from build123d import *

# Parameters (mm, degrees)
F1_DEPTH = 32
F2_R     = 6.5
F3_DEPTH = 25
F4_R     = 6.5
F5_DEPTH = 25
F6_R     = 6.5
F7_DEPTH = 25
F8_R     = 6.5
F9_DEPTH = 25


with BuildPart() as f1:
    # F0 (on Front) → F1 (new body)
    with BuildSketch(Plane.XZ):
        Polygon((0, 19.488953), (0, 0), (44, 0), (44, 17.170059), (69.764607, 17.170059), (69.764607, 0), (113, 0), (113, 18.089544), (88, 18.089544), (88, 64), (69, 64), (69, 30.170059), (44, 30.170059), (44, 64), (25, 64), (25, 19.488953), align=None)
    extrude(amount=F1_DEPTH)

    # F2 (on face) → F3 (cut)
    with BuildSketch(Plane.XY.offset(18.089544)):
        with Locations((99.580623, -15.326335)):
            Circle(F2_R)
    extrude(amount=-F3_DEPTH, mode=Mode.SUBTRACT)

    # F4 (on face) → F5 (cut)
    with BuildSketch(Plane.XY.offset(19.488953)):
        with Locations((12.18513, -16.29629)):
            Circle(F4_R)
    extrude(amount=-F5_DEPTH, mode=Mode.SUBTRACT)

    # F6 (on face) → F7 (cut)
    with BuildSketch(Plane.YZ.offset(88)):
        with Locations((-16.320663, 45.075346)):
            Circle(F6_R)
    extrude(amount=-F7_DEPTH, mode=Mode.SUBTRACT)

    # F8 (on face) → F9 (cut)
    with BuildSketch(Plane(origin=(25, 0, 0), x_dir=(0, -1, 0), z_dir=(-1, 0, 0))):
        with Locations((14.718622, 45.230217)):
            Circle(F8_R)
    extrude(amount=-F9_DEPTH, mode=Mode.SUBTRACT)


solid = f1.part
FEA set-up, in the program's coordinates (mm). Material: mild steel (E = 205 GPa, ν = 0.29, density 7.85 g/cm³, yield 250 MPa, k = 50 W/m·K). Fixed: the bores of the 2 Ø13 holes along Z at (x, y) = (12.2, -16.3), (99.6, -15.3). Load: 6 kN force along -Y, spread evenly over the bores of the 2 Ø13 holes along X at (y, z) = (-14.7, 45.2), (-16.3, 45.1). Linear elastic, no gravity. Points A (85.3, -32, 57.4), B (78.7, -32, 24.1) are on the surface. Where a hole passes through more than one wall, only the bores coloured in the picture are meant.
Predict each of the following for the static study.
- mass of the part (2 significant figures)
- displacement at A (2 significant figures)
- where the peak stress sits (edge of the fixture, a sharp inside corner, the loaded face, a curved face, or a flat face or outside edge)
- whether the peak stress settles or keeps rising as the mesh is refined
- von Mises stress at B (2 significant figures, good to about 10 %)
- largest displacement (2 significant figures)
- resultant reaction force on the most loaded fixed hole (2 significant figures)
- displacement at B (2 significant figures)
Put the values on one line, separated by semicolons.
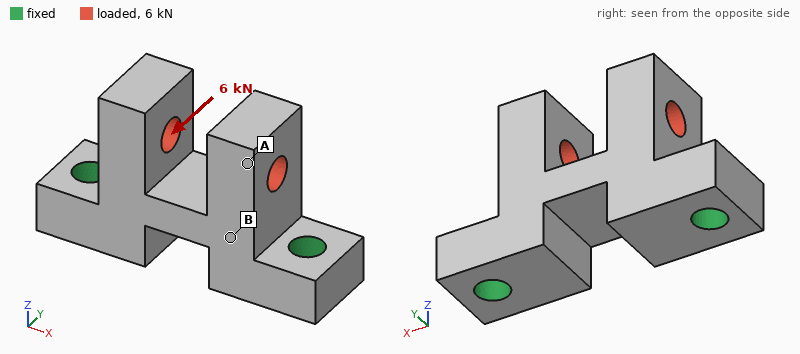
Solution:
850 g; 30 µm; edge of the fixture; keeps rising; 19 MPa; 33 µm; 3.0 kN; 12 µm
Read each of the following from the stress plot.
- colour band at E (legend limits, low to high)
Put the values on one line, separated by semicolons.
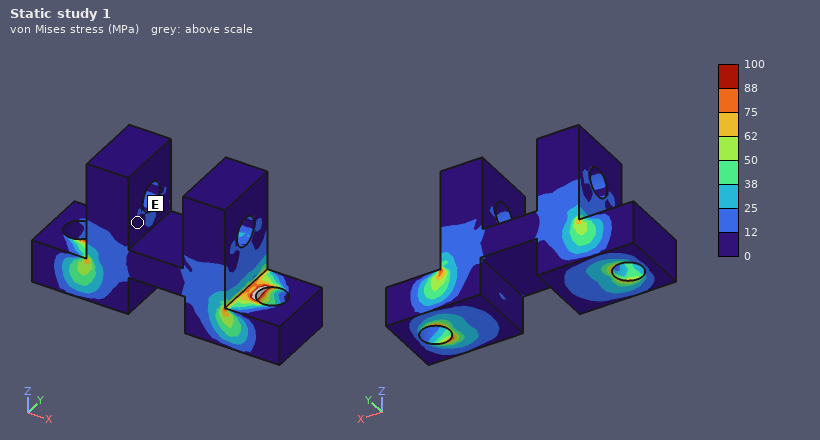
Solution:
0 to 12 MPa
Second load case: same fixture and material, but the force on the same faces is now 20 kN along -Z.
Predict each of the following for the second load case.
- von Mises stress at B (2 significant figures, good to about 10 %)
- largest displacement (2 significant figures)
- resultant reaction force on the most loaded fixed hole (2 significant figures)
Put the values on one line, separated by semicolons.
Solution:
17 MPa; 12 µm; 11 kN
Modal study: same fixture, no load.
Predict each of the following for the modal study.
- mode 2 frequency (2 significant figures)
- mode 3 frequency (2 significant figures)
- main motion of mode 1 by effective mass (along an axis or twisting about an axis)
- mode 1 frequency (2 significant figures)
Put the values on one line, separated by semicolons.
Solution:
5700 Hz; 6100 Hz; along Y; 4200 Hz
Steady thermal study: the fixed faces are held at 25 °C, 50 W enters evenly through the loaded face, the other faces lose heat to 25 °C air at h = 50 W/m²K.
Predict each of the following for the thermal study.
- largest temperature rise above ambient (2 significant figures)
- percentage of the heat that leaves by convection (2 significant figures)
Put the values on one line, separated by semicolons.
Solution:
33 K; 30 %
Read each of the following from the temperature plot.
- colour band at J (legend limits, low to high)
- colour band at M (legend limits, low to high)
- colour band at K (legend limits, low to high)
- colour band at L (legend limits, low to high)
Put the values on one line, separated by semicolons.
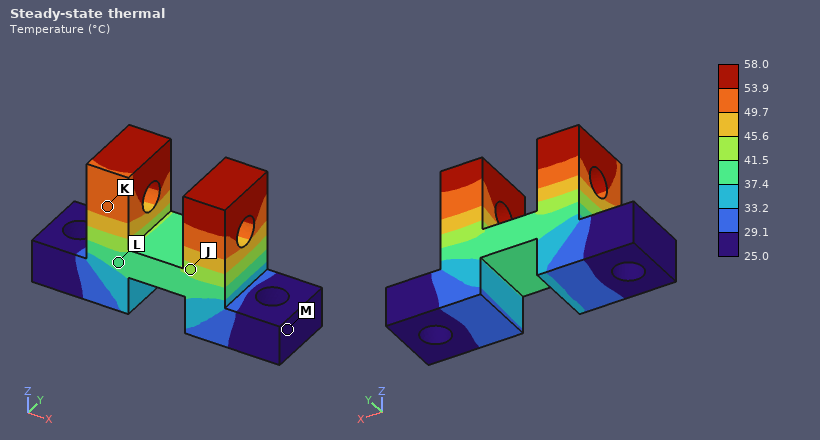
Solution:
41.5 to 45.6 °C; 25.0 to 29.1 °C; 49.7 to 53.9 °C; 37.4 to 41.5 °C
